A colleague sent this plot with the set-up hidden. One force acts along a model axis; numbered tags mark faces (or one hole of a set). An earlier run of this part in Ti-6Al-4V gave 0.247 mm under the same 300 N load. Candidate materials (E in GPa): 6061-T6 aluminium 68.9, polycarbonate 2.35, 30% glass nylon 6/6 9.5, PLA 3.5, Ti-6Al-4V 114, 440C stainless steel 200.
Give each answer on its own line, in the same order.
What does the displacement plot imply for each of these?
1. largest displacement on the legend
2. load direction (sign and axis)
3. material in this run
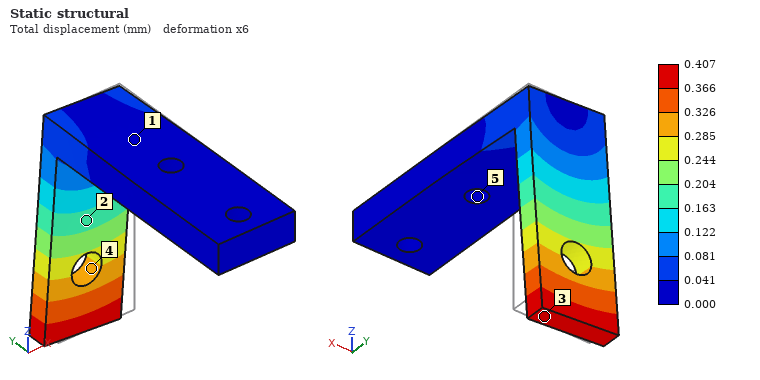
0.407 mm
-X
6061-T6 aluminium
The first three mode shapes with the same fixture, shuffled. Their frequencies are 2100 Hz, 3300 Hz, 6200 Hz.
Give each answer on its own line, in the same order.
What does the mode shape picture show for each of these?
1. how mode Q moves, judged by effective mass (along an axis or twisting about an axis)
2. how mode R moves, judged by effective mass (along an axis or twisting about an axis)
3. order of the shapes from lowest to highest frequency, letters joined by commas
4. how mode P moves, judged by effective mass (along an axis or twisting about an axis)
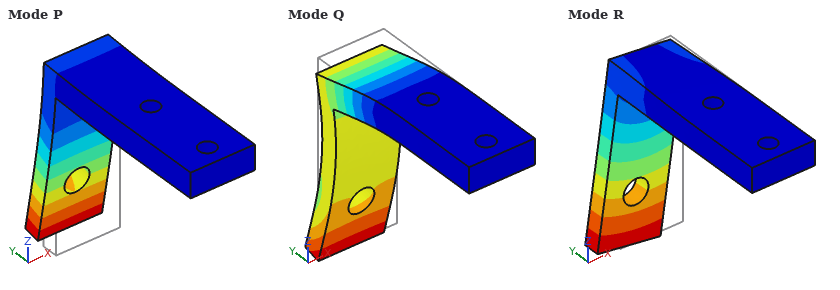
along Z
along X
P, R, Q
along Y
